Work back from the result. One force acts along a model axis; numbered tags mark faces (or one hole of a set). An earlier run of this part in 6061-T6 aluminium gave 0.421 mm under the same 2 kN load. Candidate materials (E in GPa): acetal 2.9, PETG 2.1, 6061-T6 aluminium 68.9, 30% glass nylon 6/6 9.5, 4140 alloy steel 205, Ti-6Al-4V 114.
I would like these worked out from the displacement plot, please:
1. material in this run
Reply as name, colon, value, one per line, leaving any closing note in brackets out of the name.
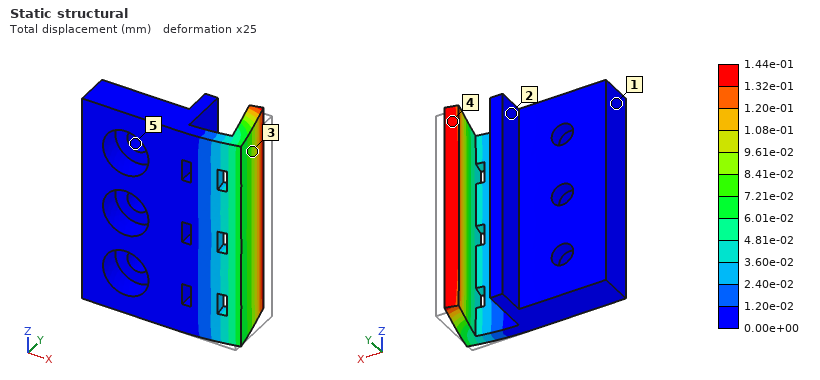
material in this run: 4140 alloy steel
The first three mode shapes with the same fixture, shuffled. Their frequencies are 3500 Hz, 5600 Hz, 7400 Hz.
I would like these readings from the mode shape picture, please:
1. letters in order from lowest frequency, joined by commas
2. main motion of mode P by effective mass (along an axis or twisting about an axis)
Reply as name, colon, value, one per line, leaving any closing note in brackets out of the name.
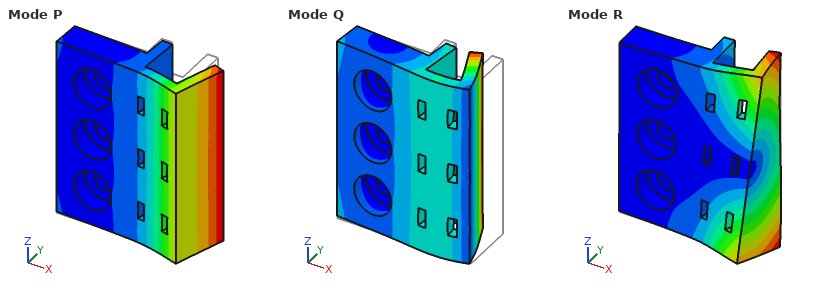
letters in order from lowest frequency, joined by commas: P, R, Q
main motion of mode P by effective mass: along Y
